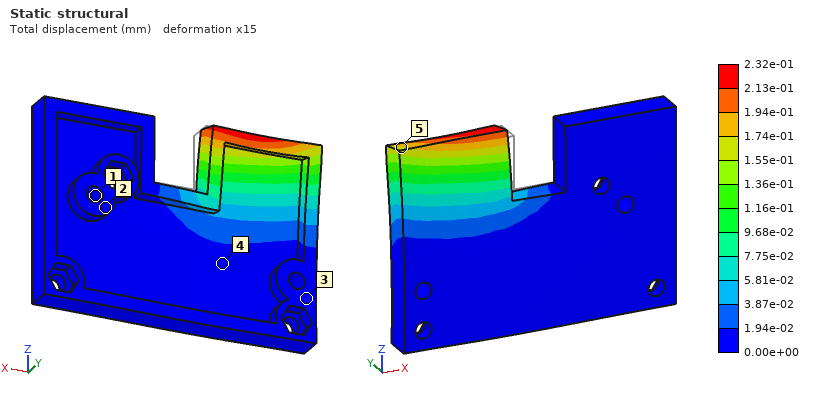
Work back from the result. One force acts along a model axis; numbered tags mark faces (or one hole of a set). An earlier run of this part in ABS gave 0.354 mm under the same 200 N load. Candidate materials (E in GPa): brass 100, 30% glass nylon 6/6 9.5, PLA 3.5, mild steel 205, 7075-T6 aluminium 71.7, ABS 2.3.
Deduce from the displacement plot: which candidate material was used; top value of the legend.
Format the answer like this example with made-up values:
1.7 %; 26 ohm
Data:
PLA; 2.32e-01 mm
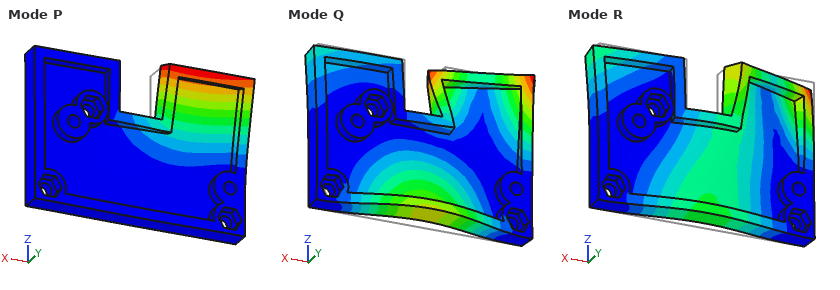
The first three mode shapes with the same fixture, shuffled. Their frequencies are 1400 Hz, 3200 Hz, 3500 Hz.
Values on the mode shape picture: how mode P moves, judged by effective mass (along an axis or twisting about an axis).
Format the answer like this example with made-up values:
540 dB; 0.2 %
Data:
along Y
